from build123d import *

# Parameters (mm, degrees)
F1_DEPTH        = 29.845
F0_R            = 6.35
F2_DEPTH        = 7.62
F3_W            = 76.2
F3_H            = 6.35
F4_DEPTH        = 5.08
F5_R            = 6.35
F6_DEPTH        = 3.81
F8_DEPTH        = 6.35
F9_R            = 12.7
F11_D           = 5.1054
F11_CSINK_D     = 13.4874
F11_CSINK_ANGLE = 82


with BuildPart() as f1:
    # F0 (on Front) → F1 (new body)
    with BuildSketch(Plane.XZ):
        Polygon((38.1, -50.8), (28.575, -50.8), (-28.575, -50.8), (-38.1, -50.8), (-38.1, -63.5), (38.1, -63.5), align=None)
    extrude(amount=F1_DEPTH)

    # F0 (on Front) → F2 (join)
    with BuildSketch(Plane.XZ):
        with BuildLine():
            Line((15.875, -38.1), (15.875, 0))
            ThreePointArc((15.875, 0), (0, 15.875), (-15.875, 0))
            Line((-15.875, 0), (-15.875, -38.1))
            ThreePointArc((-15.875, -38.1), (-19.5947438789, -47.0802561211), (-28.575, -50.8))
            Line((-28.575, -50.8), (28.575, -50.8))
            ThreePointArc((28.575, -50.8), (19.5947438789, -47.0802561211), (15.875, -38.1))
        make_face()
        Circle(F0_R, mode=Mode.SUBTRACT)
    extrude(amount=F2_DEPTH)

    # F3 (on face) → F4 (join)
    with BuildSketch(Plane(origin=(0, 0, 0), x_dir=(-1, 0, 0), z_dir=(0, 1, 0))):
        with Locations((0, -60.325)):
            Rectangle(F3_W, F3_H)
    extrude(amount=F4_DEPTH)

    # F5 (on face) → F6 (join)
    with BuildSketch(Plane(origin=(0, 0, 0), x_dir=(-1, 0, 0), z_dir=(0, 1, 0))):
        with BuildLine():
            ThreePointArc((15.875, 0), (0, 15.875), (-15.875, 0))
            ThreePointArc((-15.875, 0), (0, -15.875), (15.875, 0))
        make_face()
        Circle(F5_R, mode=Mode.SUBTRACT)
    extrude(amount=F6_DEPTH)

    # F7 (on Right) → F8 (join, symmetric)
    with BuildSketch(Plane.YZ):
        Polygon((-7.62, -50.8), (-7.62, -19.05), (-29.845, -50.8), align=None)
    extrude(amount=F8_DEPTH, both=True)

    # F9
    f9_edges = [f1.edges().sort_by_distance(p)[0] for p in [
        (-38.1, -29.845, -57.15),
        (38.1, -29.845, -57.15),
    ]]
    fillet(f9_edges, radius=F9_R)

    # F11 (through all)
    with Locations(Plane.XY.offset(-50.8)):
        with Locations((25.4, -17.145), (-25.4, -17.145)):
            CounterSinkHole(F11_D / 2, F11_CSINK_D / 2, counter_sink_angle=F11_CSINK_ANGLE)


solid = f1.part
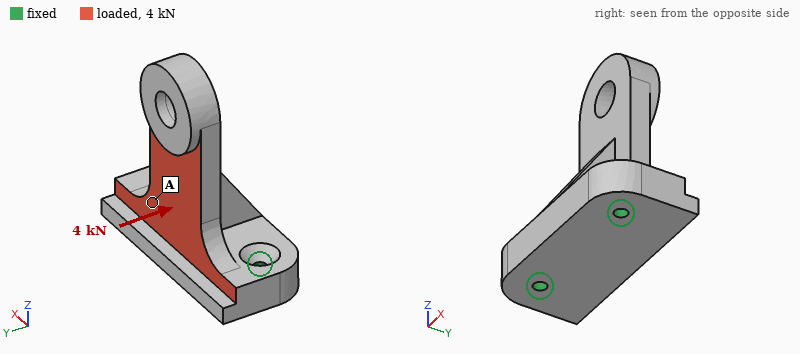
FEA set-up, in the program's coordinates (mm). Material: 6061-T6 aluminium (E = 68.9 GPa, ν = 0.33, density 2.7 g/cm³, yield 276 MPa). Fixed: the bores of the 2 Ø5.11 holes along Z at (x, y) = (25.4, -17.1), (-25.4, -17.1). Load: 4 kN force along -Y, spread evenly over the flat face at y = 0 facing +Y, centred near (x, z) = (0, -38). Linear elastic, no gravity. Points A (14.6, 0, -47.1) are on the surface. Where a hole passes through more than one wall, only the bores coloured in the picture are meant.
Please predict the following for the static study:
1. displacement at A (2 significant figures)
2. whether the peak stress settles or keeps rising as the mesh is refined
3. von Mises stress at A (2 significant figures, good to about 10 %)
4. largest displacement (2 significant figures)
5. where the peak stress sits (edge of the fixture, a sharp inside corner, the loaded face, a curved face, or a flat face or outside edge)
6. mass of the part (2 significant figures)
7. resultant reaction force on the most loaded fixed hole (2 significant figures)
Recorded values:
0.062 mm
keeps rising
27 MPa
0.30 mm
edge of the fixture
140 g
2.1 kN
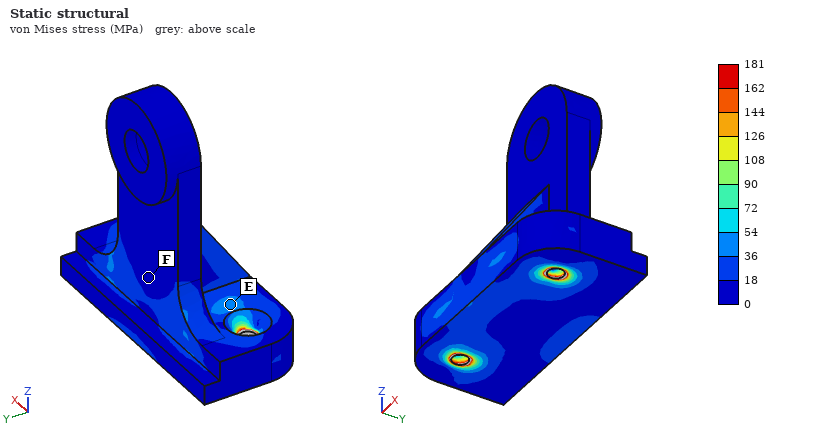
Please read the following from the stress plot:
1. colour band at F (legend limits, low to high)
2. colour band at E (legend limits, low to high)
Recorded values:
0 to 18 MPa
36 to 54 MPa
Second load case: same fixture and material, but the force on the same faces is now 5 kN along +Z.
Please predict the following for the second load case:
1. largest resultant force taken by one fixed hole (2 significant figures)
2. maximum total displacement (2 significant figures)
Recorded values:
2.6 kN
0.25 mm
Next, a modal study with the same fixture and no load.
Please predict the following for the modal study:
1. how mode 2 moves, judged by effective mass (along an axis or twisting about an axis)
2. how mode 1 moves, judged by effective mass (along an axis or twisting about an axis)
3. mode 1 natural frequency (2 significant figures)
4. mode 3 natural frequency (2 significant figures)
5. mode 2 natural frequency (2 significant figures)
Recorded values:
along X
along Y
1900 Hz
6300 Hz
4200 Hz
